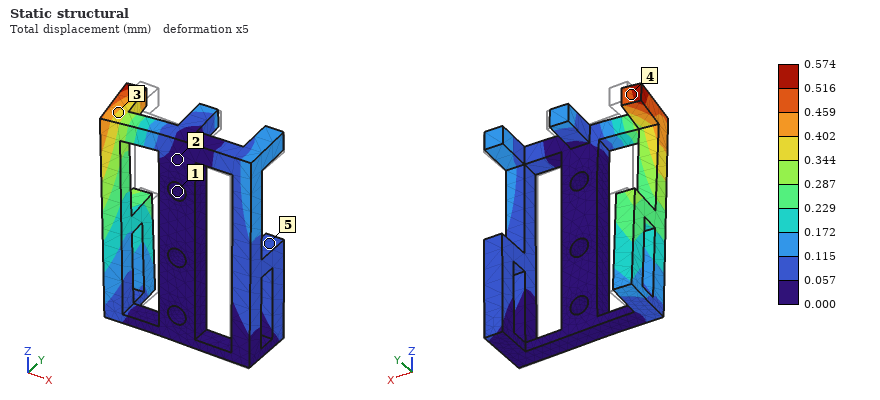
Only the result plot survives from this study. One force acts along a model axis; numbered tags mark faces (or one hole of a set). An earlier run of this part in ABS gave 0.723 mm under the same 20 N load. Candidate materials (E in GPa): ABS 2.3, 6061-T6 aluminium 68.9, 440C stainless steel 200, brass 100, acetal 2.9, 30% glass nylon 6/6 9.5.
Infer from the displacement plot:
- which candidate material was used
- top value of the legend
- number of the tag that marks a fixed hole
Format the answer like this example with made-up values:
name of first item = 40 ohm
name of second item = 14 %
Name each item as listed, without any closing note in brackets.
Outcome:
which candidate material was used = acetal
top value of the legend = 0.574 mm
number of the tag that marks a fixed hole = 1
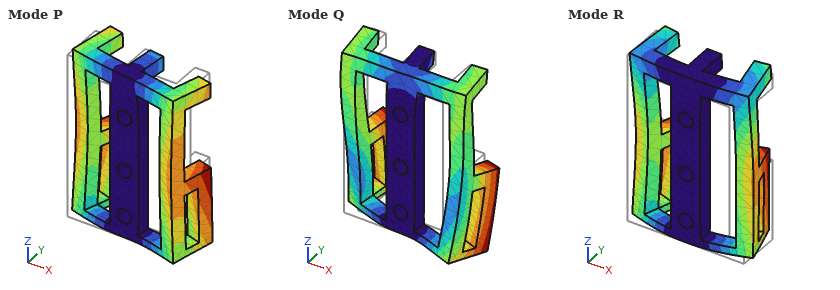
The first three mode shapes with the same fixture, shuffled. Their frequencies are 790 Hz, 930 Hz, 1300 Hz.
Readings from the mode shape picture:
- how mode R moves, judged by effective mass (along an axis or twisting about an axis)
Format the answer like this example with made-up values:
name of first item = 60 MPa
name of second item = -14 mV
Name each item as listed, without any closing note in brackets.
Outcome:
how mode R moves, judged by effective mass = along Y
